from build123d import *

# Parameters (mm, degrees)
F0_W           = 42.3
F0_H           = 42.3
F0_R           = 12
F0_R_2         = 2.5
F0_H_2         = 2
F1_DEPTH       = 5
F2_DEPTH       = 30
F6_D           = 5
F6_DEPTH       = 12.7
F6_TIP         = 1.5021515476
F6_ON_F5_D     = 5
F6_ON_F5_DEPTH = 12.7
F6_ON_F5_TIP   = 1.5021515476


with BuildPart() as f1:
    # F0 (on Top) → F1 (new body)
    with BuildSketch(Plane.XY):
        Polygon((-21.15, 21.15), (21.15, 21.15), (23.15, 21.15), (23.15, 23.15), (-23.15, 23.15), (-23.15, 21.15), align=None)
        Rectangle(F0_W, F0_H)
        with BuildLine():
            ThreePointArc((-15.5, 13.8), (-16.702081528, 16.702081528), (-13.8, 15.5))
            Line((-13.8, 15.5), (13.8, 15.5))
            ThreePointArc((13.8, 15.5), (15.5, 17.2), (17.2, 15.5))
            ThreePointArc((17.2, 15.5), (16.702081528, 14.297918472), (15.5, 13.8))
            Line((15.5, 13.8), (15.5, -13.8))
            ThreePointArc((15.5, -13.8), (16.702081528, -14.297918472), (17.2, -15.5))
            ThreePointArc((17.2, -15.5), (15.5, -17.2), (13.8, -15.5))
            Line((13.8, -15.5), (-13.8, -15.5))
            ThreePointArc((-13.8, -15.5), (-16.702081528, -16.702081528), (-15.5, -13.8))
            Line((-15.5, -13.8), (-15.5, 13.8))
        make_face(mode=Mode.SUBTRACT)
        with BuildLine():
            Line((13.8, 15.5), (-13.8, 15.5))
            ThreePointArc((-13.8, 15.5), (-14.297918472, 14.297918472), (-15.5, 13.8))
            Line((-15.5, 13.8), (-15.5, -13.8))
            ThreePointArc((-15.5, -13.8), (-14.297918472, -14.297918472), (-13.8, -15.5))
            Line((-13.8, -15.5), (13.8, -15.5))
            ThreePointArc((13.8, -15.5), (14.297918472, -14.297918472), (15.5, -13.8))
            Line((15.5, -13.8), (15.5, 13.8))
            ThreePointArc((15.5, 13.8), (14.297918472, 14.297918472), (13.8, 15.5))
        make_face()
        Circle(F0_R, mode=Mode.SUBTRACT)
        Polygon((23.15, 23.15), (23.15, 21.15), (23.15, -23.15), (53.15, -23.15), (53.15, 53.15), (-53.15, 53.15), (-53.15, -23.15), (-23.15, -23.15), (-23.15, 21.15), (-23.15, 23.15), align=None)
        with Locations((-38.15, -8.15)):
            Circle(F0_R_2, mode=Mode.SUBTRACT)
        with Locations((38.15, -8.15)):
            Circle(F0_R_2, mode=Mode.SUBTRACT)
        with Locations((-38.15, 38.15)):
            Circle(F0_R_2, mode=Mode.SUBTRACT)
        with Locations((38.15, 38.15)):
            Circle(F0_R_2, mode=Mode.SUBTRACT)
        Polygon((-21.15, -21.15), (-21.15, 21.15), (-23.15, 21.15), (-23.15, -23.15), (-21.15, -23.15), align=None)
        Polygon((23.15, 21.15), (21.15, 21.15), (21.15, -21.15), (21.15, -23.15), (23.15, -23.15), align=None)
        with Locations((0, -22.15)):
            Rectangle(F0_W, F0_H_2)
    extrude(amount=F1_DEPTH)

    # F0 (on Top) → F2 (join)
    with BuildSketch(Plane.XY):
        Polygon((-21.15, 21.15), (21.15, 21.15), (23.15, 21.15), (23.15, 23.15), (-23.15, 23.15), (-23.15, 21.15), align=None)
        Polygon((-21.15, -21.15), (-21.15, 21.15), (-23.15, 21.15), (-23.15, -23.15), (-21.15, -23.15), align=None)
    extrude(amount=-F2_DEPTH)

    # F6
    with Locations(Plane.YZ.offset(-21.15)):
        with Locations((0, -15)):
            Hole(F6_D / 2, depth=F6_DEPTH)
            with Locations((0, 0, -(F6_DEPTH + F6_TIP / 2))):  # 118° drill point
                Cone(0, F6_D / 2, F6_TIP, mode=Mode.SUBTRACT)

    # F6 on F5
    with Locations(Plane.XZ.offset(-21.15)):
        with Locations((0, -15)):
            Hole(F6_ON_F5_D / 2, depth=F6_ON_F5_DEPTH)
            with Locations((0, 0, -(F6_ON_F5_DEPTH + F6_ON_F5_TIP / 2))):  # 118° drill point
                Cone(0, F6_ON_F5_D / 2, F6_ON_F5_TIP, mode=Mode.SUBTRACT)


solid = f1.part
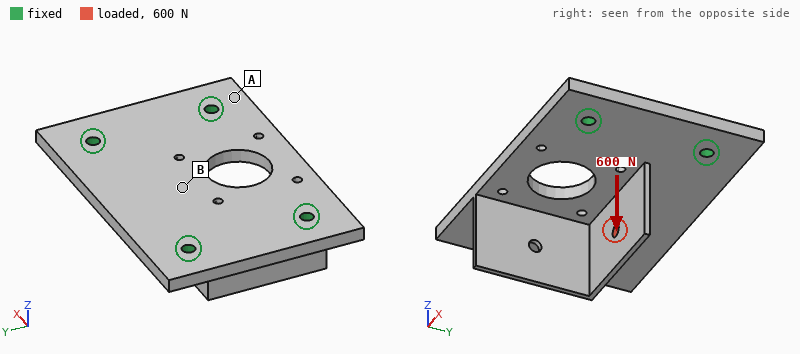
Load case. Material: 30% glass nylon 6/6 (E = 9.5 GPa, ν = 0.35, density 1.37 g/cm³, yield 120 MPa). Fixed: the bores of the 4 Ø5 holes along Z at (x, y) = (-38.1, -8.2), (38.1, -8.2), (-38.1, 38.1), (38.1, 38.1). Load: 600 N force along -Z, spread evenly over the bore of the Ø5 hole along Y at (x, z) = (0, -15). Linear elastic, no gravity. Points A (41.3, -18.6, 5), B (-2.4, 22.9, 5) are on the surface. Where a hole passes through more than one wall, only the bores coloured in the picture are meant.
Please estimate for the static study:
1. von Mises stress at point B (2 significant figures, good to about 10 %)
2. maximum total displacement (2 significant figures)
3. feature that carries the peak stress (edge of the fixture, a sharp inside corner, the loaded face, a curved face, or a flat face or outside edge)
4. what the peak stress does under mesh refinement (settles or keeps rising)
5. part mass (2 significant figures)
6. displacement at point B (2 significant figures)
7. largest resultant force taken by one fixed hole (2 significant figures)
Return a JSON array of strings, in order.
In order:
["7.8 MPa", "0.18 mm", "edge of the fixture", "keeps rising", "59 g", "0.16 mm", "210 N"]
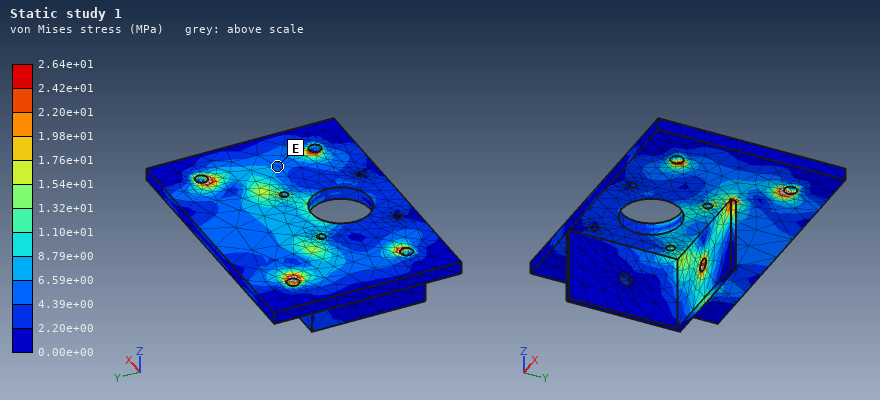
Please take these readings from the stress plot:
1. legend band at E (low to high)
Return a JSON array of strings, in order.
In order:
["4.39e+00 to 6.59e+00 MPa"]
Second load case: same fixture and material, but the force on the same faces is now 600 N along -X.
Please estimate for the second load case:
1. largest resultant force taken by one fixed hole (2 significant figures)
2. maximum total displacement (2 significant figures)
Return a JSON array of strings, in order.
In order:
["240 N", "0.15 mm"]
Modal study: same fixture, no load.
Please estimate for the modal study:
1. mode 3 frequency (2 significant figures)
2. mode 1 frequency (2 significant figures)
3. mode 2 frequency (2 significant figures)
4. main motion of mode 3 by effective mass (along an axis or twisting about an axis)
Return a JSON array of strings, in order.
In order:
["2300 Hz", "1200 Hz", "1300 Hz", "along Z"]
